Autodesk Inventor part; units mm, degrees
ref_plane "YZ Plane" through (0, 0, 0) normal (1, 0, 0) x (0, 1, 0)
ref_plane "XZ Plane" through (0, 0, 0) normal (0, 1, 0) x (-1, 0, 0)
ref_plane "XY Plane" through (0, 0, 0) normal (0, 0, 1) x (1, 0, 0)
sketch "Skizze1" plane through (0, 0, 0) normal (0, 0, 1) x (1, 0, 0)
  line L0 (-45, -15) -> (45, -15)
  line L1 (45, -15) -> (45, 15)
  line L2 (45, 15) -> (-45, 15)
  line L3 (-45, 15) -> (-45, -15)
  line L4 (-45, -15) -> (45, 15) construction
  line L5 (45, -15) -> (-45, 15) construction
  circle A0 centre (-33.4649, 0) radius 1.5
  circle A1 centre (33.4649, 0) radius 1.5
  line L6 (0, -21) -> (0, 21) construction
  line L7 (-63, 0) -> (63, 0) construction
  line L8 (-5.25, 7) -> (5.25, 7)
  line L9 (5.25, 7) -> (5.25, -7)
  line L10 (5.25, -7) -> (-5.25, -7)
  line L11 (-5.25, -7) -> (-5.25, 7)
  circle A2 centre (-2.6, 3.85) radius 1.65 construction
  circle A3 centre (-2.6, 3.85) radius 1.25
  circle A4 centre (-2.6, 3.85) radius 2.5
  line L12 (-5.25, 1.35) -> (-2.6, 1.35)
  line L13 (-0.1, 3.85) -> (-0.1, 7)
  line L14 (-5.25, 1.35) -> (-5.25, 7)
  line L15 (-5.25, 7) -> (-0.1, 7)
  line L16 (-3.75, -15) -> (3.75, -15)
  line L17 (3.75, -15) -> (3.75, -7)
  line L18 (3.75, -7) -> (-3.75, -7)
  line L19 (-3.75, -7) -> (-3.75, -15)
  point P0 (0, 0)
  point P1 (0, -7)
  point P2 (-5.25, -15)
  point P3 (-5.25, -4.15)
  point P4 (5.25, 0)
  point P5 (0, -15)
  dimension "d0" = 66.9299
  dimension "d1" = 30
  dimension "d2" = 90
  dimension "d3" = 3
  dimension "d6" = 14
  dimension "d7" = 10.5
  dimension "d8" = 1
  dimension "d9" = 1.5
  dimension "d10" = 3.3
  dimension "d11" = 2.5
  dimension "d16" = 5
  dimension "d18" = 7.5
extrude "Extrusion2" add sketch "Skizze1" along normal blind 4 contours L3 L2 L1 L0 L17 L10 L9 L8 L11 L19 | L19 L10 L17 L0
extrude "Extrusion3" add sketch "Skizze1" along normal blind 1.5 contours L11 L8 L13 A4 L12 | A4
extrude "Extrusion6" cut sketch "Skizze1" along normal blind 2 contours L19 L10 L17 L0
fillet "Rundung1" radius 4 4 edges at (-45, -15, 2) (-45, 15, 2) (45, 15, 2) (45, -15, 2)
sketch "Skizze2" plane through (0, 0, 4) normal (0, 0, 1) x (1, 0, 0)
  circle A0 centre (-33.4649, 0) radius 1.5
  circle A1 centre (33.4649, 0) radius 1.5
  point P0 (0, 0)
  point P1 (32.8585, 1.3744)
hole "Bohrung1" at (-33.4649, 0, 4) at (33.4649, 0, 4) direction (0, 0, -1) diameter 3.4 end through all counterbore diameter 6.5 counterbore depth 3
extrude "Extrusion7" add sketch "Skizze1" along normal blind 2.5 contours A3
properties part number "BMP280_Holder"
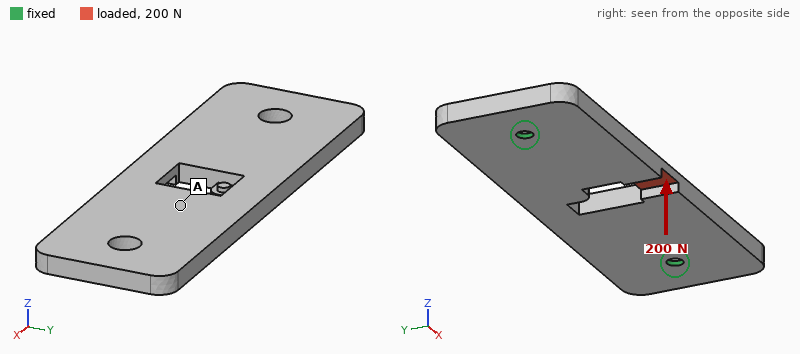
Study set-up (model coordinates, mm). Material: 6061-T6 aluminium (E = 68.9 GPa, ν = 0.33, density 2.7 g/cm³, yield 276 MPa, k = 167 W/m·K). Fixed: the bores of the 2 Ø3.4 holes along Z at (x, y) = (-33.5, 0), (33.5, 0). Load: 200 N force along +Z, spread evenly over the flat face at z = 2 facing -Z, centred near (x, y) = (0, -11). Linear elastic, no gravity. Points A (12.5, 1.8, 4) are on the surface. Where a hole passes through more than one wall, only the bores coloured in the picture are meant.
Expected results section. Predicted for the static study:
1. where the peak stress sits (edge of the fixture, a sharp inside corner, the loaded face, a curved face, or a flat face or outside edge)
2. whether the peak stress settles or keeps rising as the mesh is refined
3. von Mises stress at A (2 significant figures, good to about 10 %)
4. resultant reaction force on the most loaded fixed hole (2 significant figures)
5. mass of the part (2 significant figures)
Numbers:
edge of the fixture
keeps rising
21 MPa
610 N
27 g
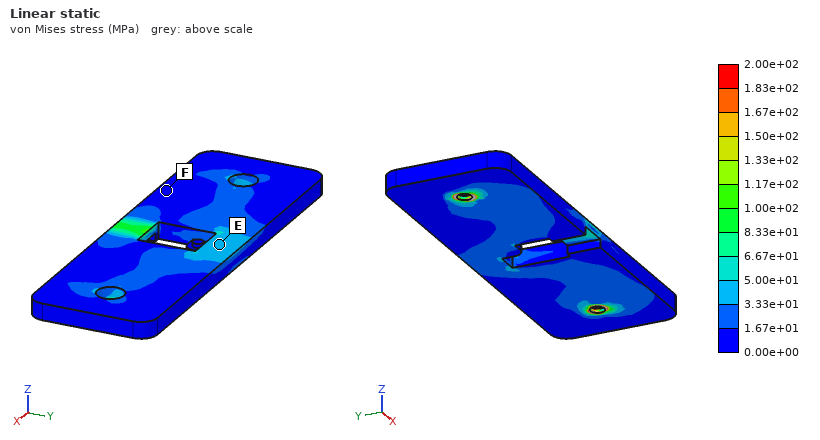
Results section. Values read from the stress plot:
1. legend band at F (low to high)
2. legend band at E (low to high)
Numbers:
0.00e+00 to 1.67e+01 MPa
3.33e+01 to 5.00e+01 MPa
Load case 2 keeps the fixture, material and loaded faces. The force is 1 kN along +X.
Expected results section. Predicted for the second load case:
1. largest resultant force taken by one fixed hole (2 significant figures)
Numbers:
530 N
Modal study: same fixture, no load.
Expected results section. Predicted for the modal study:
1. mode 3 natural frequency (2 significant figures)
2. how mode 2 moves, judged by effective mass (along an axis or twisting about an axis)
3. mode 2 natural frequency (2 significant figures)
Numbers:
4900 Hz
along Z
2700 Hz
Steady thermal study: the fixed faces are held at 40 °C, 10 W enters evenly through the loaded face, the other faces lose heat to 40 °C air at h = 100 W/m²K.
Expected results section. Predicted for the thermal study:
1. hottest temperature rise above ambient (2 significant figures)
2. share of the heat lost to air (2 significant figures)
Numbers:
20 K
33 %
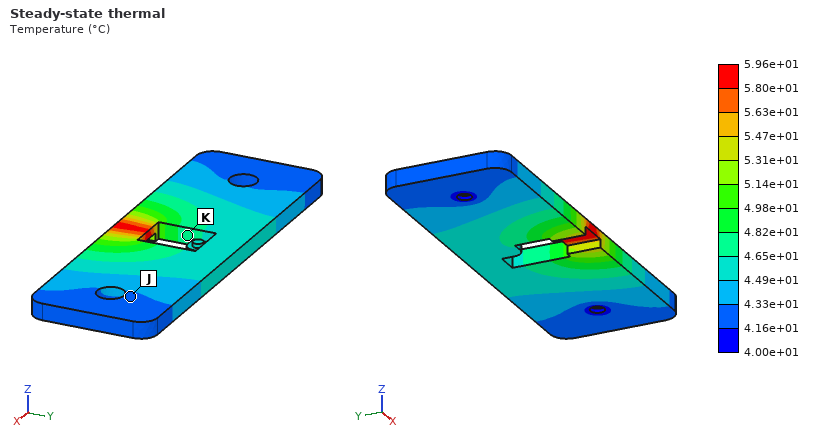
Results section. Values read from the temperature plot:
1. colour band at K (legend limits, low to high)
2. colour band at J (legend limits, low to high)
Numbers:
4.65e+01 to 4.82e+01 °C
4.16e+01 to 4.33e+01 °C
